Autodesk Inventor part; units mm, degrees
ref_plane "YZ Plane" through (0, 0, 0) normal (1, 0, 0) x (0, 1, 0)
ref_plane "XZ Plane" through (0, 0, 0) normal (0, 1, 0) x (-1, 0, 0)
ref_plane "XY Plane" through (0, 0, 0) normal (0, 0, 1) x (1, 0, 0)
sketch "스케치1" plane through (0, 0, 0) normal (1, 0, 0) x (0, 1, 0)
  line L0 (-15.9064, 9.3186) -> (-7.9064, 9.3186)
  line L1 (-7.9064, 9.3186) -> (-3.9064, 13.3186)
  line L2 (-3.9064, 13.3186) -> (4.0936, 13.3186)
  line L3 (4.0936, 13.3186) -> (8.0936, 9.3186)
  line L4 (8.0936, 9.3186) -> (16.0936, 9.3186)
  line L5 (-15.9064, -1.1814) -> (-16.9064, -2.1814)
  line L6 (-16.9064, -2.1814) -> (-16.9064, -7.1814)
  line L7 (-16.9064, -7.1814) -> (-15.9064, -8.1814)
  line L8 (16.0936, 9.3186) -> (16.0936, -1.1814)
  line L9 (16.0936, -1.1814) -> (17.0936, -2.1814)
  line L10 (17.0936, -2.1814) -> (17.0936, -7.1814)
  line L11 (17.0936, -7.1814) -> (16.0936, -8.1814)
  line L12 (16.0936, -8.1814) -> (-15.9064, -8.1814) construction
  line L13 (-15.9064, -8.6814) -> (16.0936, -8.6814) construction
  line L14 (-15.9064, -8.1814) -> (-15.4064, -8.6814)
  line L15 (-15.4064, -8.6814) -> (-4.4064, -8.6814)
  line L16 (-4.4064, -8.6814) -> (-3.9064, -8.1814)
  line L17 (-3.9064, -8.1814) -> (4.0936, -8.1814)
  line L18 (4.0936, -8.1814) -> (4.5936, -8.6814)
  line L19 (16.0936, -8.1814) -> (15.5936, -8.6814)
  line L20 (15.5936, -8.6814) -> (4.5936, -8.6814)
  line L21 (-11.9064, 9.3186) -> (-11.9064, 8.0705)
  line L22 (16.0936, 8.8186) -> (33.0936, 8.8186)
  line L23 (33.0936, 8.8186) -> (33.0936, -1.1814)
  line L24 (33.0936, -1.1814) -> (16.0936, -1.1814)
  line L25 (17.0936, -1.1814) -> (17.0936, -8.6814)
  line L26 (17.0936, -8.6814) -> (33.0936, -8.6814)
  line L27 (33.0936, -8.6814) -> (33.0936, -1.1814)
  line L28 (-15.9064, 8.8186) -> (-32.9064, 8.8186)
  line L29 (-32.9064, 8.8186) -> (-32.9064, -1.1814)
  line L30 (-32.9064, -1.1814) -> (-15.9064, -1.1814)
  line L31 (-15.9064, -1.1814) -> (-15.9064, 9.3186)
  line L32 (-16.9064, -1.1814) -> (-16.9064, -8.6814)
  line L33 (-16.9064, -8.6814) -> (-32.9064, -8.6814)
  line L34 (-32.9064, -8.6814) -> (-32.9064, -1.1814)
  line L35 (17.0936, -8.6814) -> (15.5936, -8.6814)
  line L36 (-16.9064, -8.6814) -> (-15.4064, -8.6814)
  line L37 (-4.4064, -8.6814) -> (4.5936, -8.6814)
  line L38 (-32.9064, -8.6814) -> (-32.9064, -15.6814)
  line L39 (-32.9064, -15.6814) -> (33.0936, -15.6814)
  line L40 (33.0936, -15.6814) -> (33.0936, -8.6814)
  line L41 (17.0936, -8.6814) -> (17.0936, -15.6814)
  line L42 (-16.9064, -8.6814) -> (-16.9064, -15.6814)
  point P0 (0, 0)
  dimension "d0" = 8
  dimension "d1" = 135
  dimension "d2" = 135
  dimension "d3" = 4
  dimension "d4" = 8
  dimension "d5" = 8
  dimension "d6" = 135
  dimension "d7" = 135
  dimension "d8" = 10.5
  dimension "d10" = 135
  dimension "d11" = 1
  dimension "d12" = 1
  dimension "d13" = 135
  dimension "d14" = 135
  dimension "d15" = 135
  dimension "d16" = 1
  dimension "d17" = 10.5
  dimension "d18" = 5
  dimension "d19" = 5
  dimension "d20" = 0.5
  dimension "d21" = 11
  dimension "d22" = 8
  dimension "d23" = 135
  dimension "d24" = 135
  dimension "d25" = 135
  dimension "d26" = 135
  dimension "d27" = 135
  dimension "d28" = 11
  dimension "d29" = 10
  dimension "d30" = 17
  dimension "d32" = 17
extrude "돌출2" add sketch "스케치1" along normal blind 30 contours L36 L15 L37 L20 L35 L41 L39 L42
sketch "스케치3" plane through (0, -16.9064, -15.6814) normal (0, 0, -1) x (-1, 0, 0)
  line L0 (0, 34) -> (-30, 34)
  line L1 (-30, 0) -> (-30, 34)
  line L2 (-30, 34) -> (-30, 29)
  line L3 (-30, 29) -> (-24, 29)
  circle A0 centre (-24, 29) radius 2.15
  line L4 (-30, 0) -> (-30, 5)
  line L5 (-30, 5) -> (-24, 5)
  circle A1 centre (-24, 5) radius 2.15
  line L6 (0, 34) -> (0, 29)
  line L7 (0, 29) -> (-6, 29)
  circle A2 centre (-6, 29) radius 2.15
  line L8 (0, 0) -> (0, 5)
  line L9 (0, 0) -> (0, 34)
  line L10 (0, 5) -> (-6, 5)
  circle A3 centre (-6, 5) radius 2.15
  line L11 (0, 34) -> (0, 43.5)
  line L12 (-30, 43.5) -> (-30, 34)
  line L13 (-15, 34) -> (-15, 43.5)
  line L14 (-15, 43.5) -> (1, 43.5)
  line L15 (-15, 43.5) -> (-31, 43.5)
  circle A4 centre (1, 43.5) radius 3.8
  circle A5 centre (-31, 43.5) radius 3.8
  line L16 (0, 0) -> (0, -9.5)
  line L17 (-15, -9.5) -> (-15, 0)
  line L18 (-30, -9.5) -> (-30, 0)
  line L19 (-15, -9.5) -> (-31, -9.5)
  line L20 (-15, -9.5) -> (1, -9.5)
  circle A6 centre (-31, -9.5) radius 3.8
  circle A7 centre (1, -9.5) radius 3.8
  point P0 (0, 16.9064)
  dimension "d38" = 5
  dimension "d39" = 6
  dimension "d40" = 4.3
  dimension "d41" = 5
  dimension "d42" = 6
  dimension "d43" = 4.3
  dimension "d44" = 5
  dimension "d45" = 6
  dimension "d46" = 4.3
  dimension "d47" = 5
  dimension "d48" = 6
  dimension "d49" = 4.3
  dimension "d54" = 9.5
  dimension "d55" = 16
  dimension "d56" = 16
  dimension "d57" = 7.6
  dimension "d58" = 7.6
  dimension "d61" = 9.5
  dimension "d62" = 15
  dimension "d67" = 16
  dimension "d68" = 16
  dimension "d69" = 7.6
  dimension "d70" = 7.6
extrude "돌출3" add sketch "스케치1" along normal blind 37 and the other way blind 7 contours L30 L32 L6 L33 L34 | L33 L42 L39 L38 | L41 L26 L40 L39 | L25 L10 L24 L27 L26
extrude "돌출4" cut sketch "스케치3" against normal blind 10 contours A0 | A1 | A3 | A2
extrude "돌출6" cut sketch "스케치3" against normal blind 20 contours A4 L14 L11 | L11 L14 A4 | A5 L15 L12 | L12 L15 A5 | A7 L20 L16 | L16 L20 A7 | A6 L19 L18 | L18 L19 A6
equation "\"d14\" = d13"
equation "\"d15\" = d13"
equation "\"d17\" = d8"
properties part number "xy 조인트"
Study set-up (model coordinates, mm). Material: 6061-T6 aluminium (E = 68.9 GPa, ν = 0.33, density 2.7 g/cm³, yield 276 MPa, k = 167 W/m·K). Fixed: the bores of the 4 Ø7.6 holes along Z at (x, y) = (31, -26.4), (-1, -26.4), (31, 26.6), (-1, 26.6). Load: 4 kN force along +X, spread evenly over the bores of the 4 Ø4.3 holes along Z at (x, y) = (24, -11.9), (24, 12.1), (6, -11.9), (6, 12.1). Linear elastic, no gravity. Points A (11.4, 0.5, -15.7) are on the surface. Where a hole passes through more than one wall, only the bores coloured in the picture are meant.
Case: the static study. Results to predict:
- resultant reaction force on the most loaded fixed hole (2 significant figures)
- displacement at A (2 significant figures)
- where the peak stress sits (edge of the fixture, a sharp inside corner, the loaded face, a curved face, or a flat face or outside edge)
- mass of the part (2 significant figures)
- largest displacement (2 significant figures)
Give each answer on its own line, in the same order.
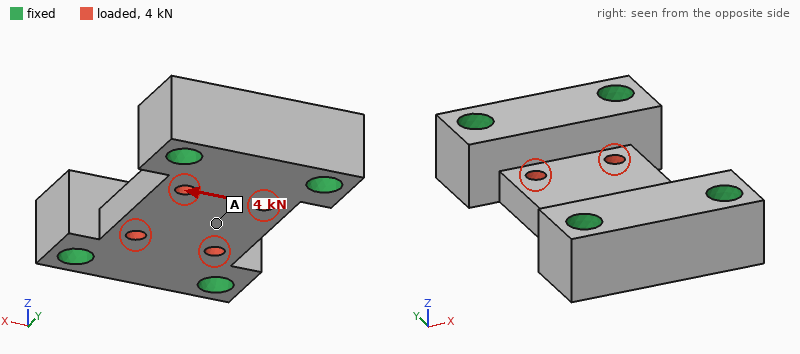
1.2 kN
5.0 µm
the loaded face
66 g
5.4 µm
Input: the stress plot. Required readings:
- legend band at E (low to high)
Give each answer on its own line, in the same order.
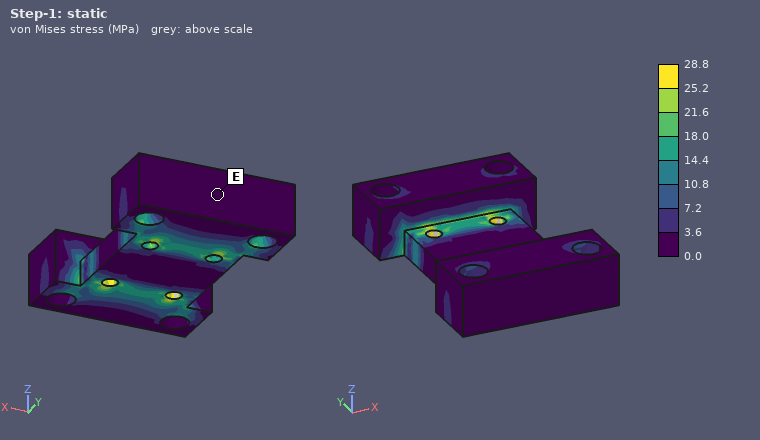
0.0 to 3.6 MPa
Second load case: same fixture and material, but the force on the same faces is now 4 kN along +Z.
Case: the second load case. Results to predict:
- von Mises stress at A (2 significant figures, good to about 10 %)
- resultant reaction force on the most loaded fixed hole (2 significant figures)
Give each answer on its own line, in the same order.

17 MPa
1.1 kN
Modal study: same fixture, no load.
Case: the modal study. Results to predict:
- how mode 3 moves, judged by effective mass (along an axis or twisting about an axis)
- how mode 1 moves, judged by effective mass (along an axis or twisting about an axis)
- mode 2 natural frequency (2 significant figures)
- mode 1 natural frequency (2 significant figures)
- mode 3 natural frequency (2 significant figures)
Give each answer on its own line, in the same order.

along X
along Z
23 kHz
17 kHz
30 kHz
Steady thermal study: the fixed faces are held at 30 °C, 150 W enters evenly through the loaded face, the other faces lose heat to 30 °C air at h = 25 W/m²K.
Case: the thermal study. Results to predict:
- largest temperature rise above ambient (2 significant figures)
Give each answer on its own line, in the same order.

30 K
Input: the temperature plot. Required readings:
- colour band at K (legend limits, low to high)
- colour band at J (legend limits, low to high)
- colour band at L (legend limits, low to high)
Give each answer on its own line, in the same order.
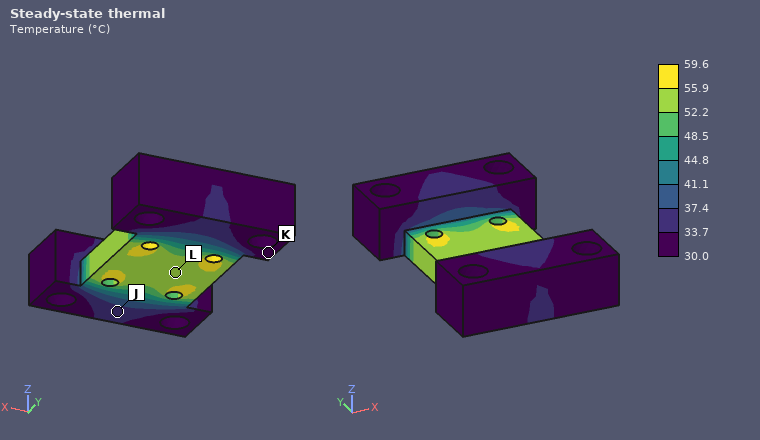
30.0 to 33.7 °C
33.7 to 37.4 °C
52.2 to 55.9 °C
